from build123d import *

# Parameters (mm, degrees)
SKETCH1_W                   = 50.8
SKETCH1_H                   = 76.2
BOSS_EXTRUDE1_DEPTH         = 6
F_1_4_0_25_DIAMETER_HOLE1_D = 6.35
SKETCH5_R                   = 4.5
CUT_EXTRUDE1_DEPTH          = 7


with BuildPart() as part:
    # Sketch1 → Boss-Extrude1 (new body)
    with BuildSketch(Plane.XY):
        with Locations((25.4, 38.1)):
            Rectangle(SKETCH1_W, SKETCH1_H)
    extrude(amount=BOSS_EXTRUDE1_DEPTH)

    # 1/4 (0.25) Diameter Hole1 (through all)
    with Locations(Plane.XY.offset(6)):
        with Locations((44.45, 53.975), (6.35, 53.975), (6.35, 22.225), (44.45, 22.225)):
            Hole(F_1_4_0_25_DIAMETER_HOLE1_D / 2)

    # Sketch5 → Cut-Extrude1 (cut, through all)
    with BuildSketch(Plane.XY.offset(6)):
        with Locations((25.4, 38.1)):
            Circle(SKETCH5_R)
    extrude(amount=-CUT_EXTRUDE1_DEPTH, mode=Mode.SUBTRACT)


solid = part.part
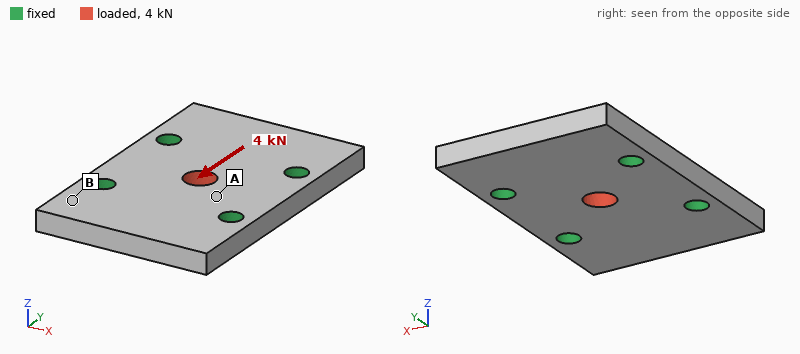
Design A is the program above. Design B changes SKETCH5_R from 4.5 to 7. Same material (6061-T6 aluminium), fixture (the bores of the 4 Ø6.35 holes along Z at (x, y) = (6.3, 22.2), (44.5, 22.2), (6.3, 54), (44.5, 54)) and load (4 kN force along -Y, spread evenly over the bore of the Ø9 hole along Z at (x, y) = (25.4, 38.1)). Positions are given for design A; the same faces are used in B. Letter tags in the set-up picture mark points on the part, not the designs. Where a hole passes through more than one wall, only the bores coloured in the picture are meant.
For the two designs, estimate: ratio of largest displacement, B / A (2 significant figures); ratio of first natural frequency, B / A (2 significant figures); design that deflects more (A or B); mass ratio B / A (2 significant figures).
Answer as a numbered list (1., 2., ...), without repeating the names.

1. 0.81
2. 0.99
3. A
4. 0.98
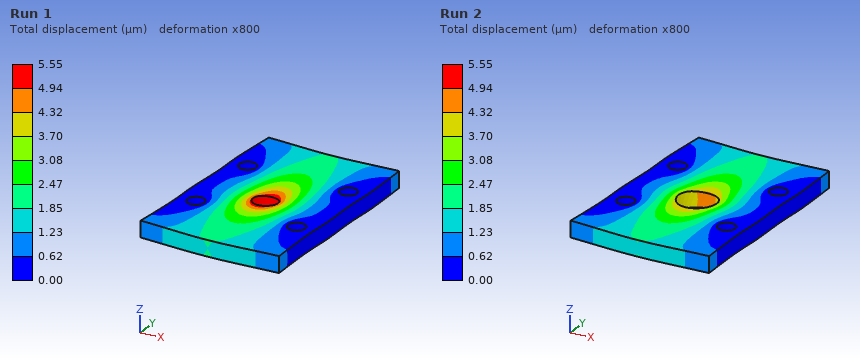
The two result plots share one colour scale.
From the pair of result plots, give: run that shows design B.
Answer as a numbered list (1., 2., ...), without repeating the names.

1. Run 2
